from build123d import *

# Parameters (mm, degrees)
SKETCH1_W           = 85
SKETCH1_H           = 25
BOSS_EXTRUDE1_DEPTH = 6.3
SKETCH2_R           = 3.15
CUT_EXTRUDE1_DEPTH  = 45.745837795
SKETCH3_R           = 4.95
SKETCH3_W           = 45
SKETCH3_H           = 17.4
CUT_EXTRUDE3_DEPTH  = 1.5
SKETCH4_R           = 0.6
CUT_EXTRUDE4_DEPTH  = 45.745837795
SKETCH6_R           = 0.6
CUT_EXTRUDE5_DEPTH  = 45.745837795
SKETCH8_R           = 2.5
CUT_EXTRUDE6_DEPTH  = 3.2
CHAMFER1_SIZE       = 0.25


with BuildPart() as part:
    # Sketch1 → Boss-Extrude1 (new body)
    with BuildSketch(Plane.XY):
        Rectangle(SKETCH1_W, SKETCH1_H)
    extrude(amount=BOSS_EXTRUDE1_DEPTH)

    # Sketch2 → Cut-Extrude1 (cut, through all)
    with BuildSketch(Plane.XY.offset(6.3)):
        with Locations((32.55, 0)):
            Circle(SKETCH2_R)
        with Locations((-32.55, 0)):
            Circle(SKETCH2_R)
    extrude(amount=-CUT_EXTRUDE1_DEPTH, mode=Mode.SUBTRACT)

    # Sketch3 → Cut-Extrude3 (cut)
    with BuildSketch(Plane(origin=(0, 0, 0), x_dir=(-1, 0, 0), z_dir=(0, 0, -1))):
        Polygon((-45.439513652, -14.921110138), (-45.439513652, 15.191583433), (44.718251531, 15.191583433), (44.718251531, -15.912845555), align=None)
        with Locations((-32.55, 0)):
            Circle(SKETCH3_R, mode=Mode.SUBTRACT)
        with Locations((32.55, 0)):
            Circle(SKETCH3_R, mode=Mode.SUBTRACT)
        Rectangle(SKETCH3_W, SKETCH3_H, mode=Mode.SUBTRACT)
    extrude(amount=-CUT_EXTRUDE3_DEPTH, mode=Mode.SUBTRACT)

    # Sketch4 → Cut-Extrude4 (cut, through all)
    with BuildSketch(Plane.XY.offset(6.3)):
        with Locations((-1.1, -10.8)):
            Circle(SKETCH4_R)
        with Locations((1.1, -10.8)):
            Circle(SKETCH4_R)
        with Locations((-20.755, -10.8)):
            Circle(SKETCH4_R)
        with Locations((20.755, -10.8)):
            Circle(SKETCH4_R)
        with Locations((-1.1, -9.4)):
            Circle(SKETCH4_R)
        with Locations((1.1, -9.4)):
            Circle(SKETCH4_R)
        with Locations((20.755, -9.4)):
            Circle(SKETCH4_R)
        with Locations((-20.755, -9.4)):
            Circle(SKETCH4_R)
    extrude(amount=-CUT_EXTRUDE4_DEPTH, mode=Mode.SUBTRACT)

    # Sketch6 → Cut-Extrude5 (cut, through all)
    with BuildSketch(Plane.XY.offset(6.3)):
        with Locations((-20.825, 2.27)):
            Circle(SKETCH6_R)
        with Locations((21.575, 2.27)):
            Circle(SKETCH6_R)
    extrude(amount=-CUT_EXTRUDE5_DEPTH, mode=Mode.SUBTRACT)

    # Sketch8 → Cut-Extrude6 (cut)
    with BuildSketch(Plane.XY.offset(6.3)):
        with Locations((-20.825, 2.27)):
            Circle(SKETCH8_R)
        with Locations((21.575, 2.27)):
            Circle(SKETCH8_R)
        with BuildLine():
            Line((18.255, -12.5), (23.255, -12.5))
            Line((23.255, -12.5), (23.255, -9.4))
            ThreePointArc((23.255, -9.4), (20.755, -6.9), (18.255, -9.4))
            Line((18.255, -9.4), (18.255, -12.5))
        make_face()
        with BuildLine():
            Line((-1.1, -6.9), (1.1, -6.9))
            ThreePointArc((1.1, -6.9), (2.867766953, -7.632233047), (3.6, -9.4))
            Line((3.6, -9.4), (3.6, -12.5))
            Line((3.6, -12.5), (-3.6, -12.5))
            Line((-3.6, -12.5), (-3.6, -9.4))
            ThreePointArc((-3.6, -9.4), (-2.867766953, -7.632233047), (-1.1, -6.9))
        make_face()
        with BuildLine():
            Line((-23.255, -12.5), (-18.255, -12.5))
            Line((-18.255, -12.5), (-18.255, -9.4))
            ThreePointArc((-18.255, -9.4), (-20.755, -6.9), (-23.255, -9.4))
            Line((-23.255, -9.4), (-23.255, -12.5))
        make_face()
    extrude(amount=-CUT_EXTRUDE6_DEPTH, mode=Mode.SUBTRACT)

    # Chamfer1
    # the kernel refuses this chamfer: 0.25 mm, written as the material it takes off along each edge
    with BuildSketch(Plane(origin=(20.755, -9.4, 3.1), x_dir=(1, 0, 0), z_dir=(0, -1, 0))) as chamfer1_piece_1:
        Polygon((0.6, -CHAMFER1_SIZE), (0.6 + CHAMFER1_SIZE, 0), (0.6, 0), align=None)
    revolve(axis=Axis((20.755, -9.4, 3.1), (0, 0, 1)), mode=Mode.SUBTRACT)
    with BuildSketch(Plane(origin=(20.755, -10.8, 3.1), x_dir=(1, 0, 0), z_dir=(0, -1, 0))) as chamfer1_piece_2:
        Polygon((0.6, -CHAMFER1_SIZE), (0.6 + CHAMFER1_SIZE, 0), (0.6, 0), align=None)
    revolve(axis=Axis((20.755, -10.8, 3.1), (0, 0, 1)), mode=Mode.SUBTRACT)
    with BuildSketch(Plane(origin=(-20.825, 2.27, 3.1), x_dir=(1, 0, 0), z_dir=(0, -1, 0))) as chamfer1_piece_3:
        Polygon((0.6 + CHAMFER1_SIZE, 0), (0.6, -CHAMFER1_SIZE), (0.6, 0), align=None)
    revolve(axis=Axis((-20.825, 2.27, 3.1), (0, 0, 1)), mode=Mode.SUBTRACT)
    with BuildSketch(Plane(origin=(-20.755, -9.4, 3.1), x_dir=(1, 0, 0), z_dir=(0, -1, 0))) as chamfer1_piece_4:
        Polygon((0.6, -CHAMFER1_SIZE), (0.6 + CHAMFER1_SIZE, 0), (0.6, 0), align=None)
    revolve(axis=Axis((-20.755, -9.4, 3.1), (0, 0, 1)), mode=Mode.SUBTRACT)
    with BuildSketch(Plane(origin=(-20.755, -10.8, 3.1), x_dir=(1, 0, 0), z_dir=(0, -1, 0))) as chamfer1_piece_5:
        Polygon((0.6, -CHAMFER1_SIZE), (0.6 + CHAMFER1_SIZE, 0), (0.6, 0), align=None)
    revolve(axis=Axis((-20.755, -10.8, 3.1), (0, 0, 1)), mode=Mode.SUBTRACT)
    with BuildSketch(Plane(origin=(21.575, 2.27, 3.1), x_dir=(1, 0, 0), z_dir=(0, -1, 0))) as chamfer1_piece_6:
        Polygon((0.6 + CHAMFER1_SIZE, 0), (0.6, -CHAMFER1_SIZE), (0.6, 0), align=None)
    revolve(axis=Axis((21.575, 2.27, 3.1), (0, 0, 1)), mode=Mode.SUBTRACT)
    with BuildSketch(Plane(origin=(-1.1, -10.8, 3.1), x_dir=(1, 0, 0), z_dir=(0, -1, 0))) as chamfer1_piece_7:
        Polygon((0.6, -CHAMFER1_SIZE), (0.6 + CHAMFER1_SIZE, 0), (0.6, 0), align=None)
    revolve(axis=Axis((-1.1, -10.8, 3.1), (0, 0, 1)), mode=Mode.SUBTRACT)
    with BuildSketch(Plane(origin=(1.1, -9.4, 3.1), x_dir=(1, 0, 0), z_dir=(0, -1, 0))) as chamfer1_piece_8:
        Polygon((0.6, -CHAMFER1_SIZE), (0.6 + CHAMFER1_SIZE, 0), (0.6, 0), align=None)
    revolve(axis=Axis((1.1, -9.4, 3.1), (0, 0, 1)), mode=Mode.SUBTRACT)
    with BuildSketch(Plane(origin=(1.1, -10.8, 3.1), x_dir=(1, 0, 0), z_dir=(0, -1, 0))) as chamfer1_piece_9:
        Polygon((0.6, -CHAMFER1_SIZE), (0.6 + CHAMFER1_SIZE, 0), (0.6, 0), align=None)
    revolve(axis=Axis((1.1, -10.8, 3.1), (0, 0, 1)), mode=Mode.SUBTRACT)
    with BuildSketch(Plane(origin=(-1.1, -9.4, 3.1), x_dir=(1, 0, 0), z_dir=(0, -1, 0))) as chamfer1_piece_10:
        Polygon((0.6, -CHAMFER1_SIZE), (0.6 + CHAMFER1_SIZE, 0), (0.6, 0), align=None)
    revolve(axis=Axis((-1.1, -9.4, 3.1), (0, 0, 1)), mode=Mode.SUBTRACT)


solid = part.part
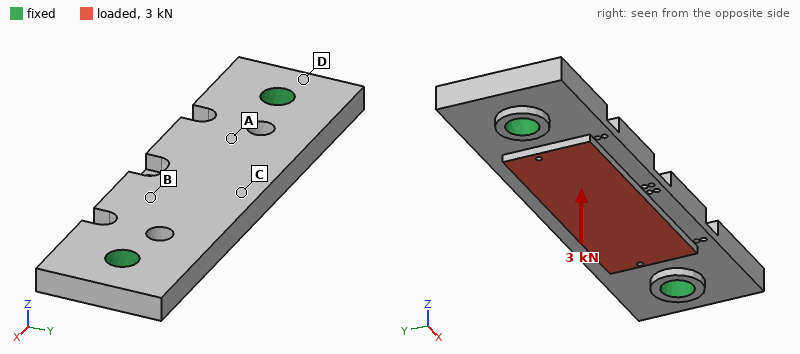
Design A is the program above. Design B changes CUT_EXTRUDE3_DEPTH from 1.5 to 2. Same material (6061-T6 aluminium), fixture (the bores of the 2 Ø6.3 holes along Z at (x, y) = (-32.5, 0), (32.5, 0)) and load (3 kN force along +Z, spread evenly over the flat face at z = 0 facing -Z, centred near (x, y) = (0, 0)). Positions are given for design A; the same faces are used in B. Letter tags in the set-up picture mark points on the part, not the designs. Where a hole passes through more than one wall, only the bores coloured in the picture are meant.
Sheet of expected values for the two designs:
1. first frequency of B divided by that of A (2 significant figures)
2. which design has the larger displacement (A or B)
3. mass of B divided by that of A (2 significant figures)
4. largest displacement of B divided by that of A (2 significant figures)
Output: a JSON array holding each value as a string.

["0.96", "B", "0.95", "1.1"]
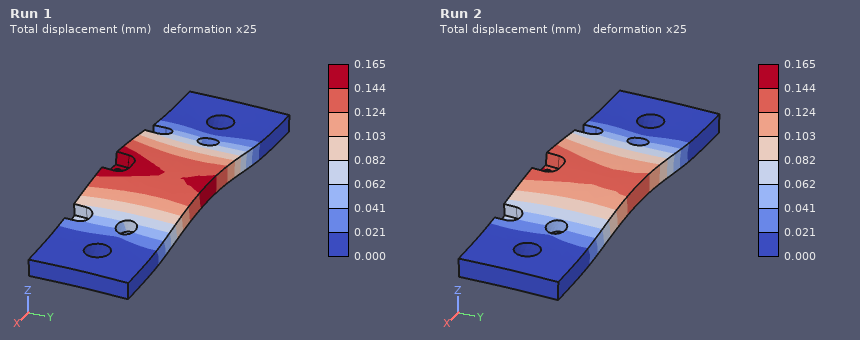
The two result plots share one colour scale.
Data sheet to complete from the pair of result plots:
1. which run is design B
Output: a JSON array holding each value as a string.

["Run 1"]
